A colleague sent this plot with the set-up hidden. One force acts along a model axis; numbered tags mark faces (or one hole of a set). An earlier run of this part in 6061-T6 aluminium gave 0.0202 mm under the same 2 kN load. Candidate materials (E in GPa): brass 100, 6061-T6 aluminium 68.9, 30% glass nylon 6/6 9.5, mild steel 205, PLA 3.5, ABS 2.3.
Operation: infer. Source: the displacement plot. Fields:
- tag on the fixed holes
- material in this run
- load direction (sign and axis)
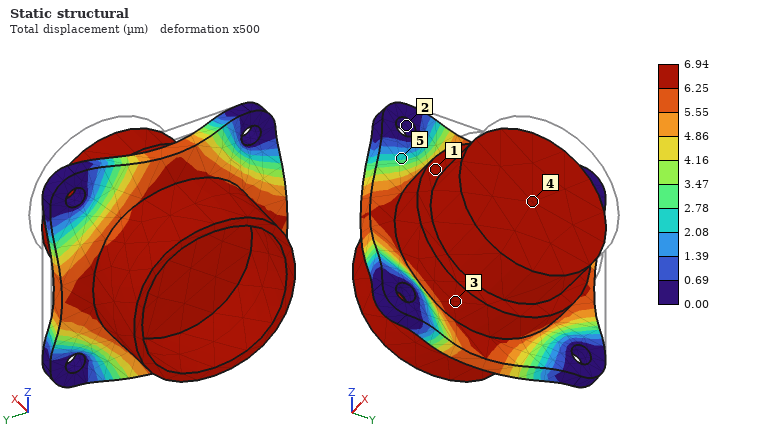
2
mild steel
-X
